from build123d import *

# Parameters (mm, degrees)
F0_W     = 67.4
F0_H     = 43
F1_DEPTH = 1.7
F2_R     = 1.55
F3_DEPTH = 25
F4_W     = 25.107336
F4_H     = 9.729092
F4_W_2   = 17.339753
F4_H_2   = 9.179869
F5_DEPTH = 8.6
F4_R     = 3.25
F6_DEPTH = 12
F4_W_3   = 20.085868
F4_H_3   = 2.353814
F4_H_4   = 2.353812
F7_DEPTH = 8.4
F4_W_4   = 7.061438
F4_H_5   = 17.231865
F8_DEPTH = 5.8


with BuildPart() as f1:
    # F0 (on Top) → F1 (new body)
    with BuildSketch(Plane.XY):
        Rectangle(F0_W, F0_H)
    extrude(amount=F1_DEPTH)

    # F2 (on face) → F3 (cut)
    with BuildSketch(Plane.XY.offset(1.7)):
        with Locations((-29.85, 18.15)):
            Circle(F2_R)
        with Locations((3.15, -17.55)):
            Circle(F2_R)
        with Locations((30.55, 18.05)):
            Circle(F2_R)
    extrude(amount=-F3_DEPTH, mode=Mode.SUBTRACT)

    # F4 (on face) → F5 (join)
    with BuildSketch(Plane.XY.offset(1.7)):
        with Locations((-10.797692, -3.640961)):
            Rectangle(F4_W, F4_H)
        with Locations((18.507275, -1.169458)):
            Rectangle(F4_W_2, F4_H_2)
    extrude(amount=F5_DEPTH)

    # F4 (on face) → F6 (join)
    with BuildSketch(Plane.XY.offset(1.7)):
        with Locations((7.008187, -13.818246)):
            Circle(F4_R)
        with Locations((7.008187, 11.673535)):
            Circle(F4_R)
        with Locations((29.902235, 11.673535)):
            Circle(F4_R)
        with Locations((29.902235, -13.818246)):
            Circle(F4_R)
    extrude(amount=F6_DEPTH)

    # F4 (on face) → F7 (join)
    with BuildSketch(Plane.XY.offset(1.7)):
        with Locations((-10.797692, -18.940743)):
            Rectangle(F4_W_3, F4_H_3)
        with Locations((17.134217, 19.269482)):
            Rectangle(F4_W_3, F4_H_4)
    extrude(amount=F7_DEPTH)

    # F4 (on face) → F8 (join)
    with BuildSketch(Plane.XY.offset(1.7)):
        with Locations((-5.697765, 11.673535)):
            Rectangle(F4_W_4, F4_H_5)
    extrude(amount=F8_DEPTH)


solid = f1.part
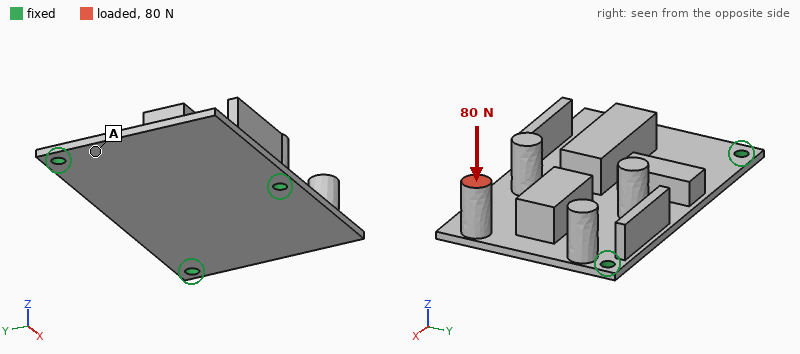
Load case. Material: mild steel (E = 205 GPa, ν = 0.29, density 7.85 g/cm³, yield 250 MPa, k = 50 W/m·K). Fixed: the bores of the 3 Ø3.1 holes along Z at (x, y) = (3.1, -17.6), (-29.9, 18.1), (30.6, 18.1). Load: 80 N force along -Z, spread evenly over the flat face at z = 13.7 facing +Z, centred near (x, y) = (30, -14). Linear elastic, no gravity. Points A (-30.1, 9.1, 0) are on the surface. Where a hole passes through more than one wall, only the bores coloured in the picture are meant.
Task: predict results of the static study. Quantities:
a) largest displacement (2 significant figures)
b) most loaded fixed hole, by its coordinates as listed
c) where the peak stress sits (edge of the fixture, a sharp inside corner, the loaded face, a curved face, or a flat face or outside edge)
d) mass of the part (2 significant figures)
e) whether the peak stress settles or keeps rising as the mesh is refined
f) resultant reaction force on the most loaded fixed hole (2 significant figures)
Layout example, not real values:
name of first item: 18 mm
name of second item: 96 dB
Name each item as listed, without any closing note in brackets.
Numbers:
largest displacement: 90 µm
most loaded fixed hole, by its coordinates as listed: (3.1, -17.6)
where the peak stress sits: edge of the fixture
mass of the part: 90 g
whether the peak stress settles or keeps rising as the mesh is refined: keeps rising
resultant reaction force on the most loaded fixed hole: 63 N
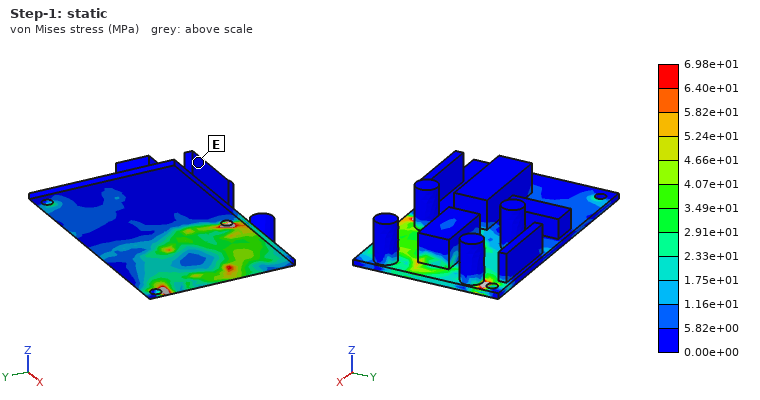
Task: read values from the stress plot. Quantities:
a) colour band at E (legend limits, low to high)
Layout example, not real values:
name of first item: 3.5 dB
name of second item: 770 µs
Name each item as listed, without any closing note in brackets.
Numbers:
colour band at E: 0.00e+00 to 5.82e+00 MPa
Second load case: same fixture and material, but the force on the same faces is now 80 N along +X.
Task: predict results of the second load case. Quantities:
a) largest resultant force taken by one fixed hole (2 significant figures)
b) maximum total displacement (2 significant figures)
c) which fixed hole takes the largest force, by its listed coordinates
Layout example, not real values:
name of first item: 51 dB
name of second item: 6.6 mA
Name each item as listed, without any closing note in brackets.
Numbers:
largest resultant force taken by one fixed hole: 51 N
maximum total displacement: 84 µm
which fixed hole takes the largest force, by its listed coordinates: (3.1, -17.6)
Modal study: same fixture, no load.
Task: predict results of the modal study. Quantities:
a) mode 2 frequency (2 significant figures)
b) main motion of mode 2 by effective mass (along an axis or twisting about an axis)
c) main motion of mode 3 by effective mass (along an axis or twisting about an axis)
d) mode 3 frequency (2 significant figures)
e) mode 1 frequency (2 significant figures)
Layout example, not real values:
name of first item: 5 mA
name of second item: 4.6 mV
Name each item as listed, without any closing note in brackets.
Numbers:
mode 2 frequency: 2100 Hz
main motion of mode 2 by effective mass: twisting about Y
main motion of mode 3 by effective mass: along Z
mode 3 frequency: 2500 Hz
mode 1 frequency: 1900 Hz
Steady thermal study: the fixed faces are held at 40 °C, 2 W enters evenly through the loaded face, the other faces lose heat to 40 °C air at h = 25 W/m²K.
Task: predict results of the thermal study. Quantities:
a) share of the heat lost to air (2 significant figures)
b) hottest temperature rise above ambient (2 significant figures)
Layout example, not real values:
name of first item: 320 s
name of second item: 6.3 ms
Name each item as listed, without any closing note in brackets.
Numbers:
share of the heat lost to air: 39 %
hottest temperature rise above ambient: 31 K
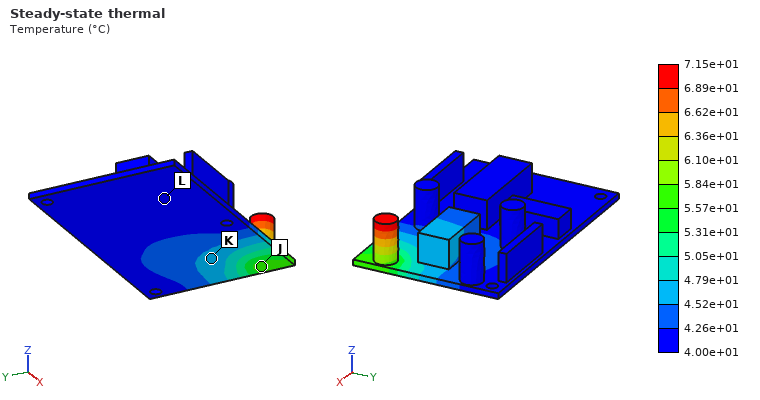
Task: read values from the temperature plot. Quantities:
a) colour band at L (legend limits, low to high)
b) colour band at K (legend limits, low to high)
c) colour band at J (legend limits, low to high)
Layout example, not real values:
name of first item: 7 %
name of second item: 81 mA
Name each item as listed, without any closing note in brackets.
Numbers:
colour band at L: 4.00e+01 to 4.26e+01 °C
colour band at K: 4.52e+01 to 4.79e+01 °C
colour band at J: 5.57e+01 to 5.84e+01 °C
